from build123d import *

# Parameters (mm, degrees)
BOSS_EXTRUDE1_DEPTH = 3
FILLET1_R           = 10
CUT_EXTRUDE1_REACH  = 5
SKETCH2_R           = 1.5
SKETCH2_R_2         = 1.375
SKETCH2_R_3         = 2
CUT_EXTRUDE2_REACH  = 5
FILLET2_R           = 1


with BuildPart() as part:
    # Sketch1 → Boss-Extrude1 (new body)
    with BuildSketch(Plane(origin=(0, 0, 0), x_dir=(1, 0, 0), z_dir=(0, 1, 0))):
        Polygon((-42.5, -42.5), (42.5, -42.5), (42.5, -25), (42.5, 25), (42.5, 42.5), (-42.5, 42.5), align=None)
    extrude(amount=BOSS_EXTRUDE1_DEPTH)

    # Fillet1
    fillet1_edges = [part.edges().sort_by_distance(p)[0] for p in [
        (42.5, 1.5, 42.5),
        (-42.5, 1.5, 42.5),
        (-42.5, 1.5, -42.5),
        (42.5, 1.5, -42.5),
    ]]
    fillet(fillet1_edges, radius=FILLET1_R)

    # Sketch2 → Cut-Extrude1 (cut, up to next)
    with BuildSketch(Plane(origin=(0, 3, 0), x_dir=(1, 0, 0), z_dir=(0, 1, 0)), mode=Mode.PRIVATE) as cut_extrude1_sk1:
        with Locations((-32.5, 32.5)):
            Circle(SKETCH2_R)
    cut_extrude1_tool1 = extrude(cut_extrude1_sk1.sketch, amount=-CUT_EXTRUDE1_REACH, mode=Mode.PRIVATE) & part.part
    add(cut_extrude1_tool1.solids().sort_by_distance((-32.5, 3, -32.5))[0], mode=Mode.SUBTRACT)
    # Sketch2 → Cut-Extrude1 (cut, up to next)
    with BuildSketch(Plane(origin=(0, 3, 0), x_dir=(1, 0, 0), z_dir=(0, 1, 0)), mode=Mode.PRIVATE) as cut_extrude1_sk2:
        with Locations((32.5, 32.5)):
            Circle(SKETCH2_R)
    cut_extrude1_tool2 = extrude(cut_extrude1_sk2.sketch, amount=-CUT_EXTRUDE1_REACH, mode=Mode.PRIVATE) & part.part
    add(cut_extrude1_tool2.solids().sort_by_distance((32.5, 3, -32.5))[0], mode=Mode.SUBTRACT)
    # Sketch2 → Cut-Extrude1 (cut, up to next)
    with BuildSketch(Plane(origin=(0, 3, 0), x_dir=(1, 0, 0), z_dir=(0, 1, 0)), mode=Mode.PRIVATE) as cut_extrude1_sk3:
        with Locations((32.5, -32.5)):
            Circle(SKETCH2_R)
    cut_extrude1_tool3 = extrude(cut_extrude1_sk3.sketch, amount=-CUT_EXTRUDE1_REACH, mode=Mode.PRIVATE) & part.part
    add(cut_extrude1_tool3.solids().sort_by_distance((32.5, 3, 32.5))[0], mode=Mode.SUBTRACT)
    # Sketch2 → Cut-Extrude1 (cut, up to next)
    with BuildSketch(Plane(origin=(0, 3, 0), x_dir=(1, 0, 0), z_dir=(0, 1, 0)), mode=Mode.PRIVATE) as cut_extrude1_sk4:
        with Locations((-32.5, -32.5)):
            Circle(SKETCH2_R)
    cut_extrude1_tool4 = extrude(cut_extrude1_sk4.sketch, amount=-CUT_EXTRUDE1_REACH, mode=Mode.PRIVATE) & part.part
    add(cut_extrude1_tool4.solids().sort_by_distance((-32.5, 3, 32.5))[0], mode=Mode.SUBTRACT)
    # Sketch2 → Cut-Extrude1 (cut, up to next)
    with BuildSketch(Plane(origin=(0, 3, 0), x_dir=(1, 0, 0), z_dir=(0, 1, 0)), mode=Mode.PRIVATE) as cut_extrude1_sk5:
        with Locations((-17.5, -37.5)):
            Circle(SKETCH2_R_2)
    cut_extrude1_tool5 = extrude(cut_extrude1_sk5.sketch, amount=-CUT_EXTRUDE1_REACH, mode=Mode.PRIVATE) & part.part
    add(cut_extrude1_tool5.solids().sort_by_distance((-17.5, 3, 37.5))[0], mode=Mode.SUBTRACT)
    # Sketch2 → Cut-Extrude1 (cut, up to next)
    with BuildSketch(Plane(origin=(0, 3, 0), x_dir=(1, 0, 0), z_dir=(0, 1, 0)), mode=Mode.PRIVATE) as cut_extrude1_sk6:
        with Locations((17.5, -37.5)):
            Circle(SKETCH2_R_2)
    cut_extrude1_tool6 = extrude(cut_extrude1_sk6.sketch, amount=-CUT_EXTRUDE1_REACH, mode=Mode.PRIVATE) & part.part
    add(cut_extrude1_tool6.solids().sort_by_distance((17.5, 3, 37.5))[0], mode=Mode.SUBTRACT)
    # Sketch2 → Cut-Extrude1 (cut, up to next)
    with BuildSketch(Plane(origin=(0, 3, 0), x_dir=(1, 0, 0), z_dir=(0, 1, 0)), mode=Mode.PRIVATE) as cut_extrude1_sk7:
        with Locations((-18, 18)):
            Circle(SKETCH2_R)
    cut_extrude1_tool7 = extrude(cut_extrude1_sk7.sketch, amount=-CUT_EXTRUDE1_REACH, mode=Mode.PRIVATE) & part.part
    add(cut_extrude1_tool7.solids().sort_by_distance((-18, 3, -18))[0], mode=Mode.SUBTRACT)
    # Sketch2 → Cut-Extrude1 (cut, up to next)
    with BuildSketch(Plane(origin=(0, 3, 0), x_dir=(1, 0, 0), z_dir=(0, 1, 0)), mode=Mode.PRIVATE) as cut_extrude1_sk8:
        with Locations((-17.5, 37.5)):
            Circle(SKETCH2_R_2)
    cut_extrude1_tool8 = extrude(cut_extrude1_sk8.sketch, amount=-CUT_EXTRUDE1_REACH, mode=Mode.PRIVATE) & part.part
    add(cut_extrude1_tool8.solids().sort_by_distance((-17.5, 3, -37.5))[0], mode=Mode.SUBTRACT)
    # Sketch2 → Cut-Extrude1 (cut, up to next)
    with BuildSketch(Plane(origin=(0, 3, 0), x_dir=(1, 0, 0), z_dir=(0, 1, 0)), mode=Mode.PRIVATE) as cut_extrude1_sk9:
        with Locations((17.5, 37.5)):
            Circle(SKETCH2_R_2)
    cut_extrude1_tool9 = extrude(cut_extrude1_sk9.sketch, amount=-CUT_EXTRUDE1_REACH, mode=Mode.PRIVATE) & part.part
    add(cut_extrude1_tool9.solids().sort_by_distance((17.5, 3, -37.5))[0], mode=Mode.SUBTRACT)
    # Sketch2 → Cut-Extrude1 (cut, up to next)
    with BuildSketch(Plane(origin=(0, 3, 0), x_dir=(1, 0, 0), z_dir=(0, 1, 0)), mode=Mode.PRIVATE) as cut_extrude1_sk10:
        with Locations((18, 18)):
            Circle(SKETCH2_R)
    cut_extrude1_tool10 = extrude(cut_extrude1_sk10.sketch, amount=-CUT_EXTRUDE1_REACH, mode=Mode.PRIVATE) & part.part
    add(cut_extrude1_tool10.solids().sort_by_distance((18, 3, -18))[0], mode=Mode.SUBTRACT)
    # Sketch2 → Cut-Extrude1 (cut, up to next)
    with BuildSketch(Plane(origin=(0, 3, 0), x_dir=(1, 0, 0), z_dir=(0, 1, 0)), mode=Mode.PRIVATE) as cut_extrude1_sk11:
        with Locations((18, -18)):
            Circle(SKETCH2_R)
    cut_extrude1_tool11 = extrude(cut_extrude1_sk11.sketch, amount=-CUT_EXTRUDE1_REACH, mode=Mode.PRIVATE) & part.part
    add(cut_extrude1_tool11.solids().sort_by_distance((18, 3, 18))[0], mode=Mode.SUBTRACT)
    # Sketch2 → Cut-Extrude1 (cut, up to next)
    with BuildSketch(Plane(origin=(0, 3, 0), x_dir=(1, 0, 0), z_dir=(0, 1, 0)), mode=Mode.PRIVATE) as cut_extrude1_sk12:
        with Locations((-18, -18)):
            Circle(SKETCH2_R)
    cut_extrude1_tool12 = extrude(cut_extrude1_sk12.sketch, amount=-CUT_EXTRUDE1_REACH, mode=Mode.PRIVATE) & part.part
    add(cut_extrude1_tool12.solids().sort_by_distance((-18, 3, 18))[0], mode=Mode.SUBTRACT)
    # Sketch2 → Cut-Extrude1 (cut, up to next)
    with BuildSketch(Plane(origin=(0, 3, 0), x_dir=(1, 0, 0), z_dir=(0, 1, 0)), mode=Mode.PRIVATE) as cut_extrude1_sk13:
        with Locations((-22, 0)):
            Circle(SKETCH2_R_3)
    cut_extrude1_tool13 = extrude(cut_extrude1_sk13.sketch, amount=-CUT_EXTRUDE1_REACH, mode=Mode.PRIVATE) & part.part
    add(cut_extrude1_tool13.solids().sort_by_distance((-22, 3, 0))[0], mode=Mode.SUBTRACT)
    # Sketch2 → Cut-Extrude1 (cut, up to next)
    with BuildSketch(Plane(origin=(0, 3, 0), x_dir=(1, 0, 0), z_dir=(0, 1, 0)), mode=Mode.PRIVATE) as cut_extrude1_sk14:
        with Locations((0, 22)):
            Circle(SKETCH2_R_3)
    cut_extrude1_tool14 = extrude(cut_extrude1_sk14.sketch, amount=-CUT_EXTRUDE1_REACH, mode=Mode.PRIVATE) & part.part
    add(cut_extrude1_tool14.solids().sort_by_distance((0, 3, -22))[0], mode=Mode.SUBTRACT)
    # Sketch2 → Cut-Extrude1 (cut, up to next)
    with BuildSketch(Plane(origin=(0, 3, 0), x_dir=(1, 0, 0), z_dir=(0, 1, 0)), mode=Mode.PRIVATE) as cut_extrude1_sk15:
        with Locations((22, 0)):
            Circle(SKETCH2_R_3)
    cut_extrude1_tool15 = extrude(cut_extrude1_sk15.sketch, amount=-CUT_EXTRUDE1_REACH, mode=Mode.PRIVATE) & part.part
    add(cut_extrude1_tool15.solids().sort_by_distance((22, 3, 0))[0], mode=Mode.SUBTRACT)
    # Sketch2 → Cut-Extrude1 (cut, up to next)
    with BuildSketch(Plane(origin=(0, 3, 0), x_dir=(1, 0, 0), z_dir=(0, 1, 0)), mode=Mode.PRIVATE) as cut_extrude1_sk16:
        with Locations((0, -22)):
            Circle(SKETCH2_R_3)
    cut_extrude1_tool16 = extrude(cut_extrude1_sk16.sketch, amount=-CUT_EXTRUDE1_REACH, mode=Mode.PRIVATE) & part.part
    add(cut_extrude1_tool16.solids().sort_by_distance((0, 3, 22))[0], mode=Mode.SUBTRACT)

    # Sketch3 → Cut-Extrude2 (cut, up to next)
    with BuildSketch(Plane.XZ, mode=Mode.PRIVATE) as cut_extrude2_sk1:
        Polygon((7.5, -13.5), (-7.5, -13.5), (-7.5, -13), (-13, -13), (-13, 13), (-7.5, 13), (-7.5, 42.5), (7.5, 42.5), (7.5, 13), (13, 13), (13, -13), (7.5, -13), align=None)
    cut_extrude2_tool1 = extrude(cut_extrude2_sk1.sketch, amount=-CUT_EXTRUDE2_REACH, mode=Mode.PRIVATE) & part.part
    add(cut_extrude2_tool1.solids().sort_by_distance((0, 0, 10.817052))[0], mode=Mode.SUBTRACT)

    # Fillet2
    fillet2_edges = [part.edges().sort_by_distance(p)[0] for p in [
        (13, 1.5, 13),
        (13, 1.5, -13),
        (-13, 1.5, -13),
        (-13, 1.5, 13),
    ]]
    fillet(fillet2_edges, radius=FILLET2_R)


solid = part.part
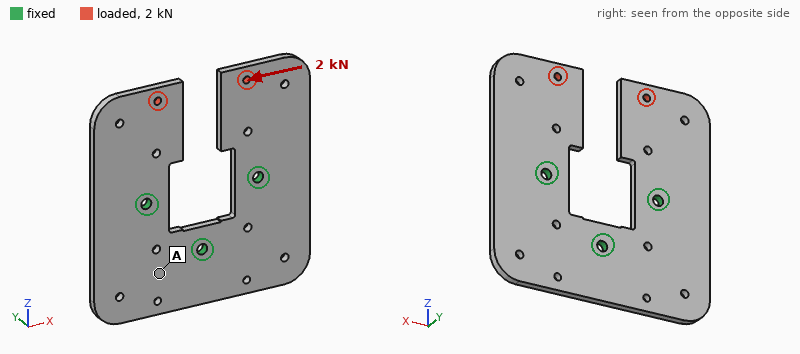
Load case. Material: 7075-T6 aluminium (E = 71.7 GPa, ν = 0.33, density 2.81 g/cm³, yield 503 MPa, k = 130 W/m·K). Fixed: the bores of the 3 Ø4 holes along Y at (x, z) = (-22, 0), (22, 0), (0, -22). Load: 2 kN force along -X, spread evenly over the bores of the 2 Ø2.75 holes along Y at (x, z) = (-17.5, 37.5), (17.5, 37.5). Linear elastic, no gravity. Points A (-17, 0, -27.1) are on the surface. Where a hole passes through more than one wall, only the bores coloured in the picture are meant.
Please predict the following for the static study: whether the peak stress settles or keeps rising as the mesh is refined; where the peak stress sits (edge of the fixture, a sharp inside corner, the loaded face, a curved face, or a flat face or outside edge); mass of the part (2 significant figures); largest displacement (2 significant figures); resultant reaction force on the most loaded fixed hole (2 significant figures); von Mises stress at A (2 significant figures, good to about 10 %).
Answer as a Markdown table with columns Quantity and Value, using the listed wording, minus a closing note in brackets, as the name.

| Quantity | Value |
|---|---|
| whether the peak stress settles or keeps rising as the mesh is refined | keeps rising |
| where the peak stress sits | edge of the fixture |
| mass of the part | 50 g |
| largest displacement | 0.15 mm |
| resultant reaction force on the most loaded fixed hole | 2.2 kN |
| von Mises stress at A | 20 MPa |
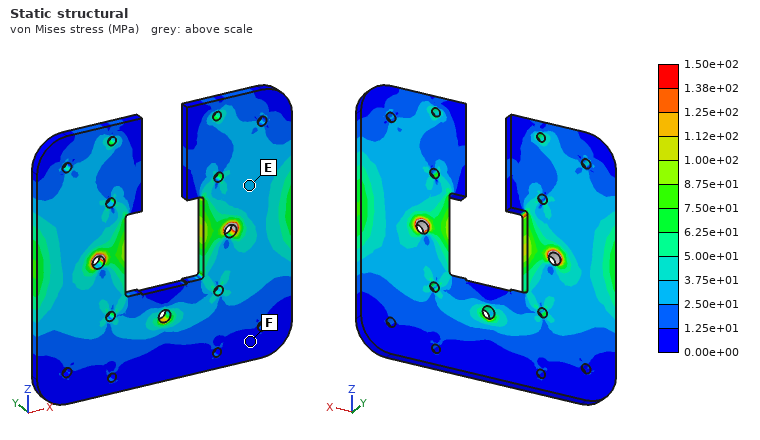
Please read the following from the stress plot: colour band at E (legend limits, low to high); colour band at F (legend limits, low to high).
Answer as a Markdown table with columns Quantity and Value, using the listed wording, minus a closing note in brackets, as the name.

| Quantity | Value |
|---|---|
| colour band at E | 2.50e+01 to 3.75e+01 MPa |
| colour band at F | 0.00e+00 to 1.25e+01 MPa |
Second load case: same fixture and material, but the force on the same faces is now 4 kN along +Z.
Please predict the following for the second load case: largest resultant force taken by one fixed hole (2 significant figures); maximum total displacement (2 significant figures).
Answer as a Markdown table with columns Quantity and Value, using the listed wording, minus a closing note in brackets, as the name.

| Quantity | Value |
|---|---|
| largest resultant force taken by one fixed hole | 2.0 kN |
| maximum total displacement | 57 µm |
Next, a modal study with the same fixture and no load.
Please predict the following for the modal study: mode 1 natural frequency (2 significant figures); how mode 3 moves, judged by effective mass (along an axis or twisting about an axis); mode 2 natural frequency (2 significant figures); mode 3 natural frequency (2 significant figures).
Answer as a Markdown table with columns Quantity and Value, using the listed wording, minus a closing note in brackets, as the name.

| Quantity | Value |
|---|---|
| mode 1 natural frequency | 1200 Hz |
| how mode 3 moves, judged by effective mass | twisting about Z |
| mode 2 natural frequency | 1200 Hz |
| mode 3 natural frequency | 2200 Hz |
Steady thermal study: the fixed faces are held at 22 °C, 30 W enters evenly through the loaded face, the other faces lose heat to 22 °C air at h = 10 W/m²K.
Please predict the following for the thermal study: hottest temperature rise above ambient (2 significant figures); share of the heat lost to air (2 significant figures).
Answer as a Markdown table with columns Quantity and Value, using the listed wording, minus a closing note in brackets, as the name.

| Quantity | Value |
|---|---|
| hottest temperature rise above ambient | 64 K |
| share of the heat lost to air | 7.4 % |
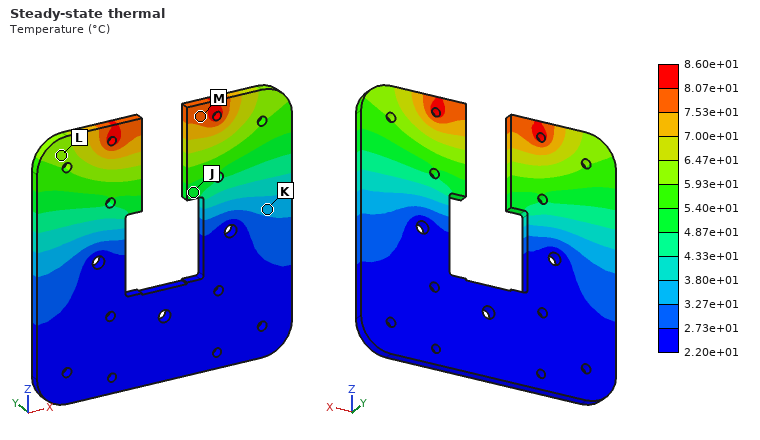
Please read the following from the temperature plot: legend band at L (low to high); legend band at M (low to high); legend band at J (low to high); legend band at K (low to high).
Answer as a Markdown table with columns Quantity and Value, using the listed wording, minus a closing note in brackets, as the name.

| Quantity | Value |
|---|---|
| legend band at L | 5.93e+01 to 6.47e+01 °C |
| legend band at M | 7.53e+01 to 8.07e+01 °C |
| legend band at J | 4.87e+01 to 5.40e+01 °C |
| legend band at K | 3.27e+01 to 3.80e+01 °C |
